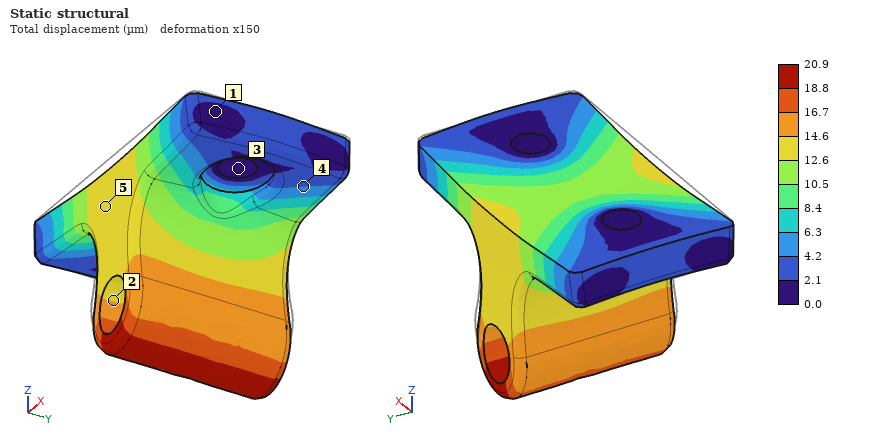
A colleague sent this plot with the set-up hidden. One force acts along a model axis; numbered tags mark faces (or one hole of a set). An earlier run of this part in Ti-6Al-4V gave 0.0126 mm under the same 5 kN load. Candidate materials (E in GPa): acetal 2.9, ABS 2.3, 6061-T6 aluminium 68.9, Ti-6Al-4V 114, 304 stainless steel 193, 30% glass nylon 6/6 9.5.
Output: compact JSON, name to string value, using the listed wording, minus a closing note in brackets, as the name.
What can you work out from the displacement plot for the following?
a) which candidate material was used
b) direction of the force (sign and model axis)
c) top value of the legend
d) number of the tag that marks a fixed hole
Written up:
{"which candidate material was used": "6061-T6 aluminium", "direction of the force": "-Z", "top value of the legend": "20.9 µm", "number of the tag that marks a fixed hole": "3"}
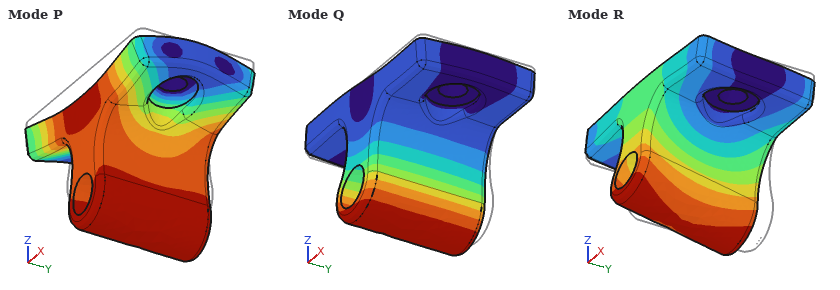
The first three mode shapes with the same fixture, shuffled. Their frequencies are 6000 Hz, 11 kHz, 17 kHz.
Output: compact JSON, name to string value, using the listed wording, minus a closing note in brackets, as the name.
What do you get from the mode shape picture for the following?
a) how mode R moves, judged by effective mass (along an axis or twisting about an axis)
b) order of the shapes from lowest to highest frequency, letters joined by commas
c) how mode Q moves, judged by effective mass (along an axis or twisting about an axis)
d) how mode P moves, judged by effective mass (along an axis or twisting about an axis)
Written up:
{"how mode R moves, judged by effective mass": "along Y", "order of the shapes from lowest to highest frequency, letters joined by commas": "R, Q, P", "how mode Q moves, judged by effective mass": "along X", "how mode P moves, judged by effective mass": "along Z"}
